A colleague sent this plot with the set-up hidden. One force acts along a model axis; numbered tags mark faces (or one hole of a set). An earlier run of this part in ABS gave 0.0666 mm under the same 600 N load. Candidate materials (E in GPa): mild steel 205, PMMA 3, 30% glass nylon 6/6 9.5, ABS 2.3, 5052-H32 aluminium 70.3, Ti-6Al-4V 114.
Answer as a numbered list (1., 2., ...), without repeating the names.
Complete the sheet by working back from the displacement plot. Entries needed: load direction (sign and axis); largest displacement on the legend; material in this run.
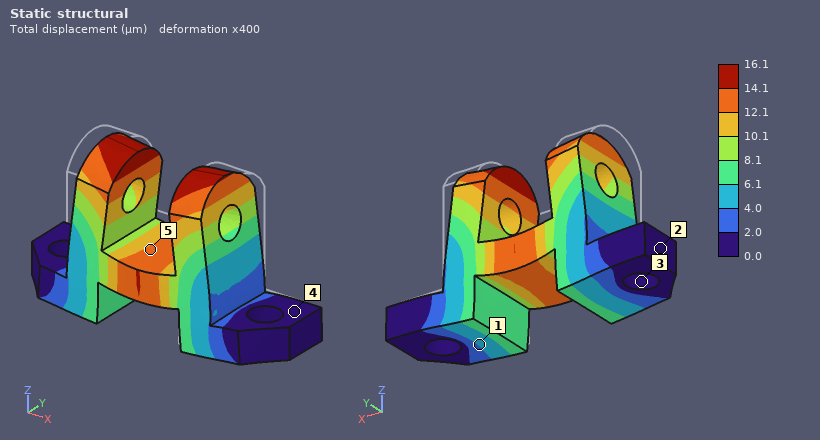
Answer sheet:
1. -Z
2. 16.1 µm
3. 30% glass nylon 6/6
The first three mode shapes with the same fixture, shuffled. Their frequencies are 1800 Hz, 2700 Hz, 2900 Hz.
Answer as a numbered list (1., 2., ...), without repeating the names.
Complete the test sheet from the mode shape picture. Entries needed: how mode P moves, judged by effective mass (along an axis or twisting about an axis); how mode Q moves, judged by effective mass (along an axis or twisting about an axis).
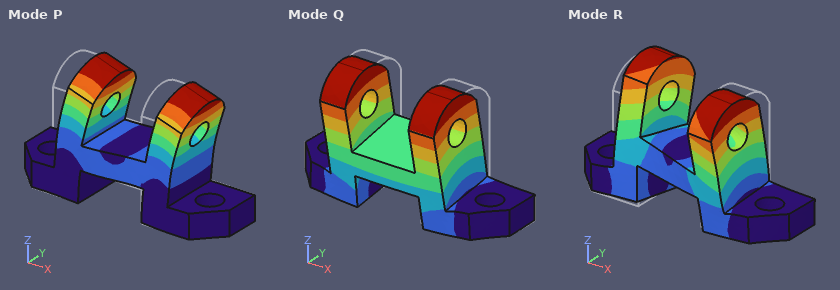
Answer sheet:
1. along X
2. along Y
